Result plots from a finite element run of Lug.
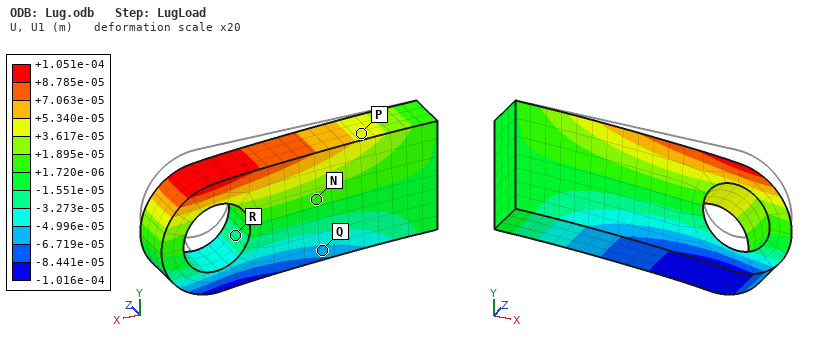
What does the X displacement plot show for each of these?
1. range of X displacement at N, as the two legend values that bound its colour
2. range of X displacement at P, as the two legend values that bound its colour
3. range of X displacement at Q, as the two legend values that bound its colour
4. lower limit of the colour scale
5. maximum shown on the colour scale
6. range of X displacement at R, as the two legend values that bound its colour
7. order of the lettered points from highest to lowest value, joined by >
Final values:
+1.720e-06 to +1.895e-05 m
+3.617e-05 to +5.340e-05 m
-6.719e-05 to -4.996e-05 m
-1.016e-04 m
+1.051e-04 m
-3.273e-05 to -1.551e-05 m
P > N > R > Q
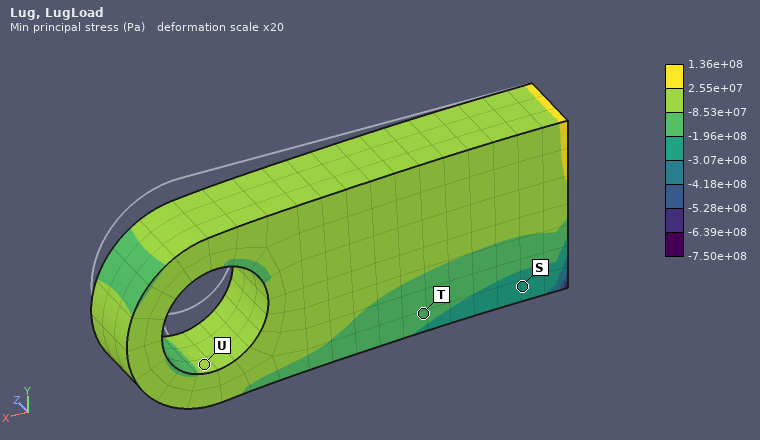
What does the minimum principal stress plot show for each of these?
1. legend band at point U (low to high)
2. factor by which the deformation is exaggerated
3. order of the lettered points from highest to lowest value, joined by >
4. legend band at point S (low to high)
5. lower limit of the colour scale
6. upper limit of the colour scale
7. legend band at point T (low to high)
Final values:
-8.53e+07 to 2.55e+07 Pa
20
U > T > S
-3.07e+08 to -1.96e+08 Pa
-7.50e+08 Pa
1.36e+08 Pa
-1.96e+08 to -8.53e+07 Pa
